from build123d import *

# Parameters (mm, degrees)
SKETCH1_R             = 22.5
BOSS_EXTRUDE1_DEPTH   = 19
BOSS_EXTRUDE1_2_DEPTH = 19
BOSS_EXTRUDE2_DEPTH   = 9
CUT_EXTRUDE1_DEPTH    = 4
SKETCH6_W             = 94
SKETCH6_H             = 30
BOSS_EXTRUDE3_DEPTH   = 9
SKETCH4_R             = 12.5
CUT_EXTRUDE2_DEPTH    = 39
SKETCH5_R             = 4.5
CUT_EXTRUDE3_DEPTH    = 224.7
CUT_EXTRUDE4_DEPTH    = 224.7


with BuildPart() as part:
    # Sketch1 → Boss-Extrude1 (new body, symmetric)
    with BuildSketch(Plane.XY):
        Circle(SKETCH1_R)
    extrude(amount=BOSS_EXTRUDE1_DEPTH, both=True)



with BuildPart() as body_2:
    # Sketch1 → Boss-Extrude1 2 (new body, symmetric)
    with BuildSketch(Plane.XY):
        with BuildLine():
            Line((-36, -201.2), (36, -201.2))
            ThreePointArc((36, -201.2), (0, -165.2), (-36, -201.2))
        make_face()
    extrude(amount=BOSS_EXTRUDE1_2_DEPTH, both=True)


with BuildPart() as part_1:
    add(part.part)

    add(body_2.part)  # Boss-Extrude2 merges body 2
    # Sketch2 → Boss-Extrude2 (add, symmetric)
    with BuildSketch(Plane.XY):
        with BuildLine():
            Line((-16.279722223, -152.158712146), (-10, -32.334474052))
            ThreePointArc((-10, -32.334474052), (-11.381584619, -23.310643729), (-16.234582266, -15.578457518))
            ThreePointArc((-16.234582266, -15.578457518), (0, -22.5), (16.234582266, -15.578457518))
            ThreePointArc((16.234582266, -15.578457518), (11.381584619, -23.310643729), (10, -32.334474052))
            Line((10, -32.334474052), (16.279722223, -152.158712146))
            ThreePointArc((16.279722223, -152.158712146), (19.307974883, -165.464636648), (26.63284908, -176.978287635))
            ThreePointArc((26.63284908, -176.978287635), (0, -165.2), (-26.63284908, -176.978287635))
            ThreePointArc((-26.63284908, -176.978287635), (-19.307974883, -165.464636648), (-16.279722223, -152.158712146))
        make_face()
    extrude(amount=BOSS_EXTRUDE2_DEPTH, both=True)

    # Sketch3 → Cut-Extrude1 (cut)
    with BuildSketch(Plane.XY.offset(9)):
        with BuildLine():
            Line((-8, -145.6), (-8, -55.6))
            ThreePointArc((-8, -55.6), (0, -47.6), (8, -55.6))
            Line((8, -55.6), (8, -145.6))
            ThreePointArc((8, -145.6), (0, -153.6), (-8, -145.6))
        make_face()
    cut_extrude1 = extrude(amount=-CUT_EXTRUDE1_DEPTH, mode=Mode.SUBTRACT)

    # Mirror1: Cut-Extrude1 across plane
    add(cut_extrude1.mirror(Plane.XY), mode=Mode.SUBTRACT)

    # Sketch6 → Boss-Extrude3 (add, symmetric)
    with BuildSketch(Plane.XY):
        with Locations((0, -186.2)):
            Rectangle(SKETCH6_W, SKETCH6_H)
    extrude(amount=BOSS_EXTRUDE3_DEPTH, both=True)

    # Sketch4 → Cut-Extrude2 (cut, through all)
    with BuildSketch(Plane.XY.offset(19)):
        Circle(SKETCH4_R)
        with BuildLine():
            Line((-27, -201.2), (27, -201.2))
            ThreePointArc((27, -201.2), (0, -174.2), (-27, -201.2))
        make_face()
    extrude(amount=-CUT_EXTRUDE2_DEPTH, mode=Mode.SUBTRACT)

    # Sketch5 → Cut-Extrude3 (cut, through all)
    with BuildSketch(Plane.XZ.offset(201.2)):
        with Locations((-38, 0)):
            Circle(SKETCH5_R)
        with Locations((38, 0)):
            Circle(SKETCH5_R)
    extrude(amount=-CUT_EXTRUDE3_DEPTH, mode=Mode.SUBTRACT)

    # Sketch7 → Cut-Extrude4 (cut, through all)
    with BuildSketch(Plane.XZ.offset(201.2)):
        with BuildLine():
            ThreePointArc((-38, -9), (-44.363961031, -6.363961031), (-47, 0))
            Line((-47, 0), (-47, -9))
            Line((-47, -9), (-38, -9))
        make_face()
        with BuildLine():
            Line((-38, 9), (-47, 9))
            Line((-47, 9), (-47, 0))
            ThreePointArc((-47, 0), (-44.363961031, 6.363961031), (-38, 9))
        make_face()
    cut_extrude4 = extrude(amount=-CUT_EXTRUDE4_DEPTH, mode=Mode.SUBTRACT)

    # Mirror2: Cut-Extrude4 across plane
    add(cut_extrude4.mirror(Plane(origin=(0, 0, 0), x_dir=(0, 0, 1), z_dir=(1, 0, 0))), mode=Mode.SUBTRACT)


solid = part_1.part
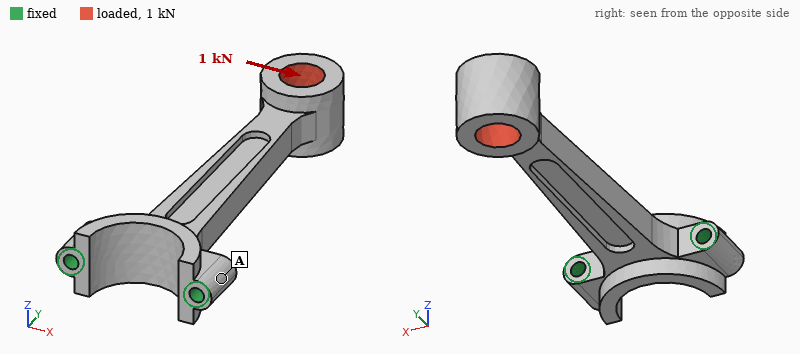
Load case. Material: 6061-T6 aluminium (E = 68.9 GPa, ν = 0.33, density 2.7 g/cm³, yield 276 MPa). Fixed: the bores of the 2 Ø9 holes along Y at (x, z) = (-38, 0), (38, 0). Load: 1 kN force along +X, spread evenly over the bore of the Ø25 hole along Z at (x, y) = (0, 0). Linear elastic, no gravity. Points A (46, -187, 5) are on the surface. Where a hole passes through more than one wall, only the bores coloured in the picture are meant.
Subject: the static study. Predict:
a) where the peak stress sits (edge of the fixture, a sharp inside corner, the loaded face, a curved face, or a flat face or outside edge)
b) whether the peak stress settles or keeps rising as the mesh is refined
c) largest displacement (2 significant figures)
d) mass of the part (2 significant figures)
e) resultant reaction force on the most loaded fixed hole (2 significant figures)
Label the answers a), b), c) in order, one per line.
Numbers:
a) edge of the fixture
b) keeps rising
c) 0.98 mm
d) 390 g
e) 3.9 kN
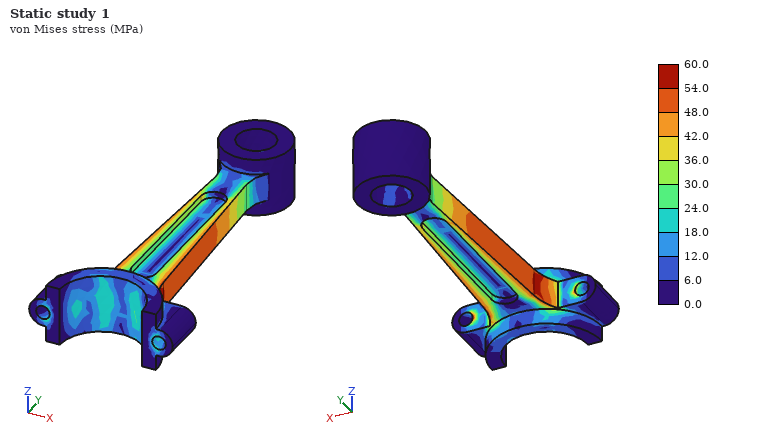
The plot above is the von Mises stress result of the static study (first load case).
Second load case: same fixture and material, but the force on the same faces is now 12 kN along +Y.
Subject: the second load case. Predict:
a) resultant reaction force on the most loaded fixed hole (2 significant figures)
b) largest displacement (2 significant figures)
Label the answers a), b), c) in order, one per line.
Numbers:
a) 7.5 kN
b) 0.11 mm
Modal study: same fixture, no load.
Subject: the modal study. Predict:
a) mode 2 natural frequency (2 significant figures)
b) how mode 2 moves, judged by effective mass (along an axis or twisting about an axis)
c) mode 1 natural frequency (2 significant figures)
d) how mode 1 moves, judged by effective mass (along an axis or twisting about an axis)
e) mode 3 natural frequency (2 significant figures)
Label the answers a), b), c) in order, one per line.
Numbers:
a) 480 Hz
b) along X
c) 240 Hz
d) along Z
e) 1200 Hz
